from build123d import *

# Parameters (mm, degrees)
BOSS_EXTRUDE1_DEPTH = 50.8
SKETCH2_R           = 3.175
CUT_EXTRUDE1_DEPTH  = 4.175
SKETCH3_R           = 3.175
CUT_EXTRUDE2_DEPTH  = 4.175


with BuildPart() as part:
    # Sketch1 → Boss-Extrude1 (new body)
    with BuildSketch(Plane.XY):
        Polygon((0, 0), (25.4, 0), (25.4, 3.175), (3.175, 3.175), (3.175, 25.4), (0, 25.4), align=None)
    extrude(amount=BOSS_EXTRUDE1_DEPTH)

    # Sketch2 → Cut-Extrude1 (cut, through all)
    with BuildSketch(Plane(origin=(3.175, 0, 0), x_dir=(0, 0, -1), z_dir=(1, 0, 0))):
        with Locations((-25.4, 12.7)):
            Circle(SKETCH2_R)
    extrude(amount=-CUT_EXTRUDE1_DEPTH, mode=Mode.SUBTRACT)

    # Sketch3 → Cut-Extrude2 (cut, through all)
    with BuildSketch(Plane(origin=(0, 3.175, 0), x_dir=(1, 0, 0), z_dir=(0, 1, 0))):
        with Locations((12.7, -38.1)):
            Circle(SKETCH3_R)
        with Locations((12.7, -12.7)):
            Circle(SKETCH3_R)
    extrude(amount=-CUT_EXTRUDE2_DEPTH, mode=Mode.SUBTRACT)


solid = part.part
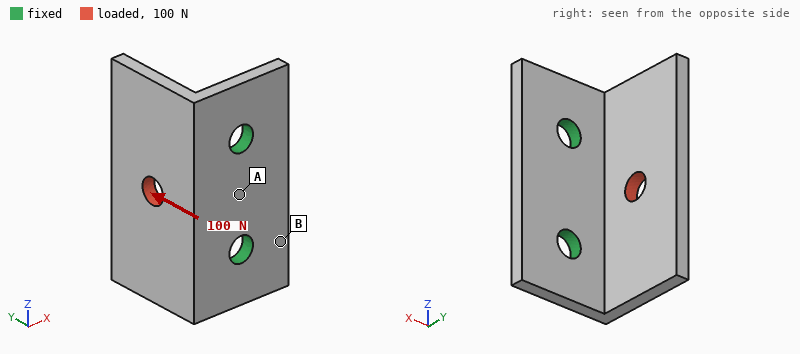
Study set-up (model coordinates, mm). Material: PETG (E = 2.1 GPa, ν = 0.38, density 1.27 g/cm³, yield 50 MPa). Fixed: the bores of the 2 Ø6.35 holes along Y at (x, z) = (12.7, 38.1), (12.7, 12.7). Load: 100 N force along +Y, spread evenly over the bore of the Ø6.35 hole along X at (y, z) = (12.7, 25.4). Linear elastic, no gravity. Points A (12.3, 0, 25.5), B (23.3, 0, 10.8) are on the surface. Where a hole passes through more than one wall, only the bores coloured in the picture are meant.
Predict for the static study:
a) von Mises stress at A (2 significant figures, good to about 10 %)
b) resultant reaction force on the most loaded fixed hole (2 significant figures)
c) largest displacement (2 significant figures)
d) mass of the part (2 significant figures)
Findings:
3.0 MPa
51 N
0.42 mm
9.4 g
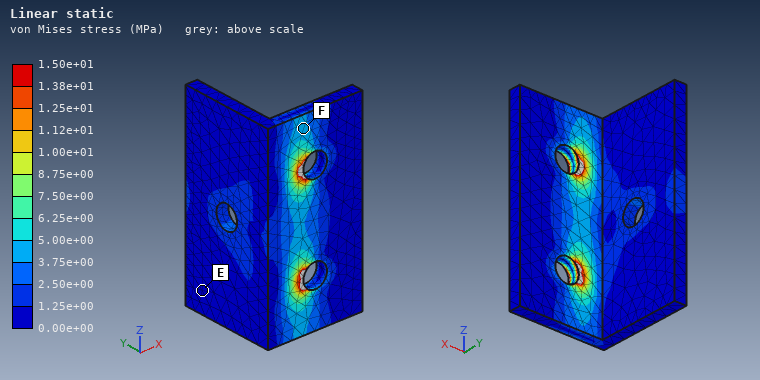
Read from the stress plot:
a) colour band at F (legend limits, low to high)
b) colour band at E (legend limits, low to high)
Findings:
3.75e+00 to 5.00e+00 MPa
0.00e+00 to 1.25e+00 MPa
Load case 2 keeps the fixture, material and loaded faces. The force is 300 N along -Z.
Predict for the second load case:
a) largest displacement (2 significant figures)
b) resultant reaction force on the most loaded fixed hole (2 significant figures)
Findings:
0.65 mm
210 N
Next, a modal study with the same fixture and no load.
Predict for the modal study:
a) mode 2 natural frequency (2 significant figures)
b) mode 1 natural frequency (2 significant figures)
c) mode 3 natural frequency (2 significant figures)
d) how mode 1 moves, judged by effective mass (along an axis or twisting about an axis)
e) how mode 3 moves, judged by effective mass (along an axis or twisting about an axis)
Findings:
1200 Hz
740 Hz
2100 Hz
along X
along Z
